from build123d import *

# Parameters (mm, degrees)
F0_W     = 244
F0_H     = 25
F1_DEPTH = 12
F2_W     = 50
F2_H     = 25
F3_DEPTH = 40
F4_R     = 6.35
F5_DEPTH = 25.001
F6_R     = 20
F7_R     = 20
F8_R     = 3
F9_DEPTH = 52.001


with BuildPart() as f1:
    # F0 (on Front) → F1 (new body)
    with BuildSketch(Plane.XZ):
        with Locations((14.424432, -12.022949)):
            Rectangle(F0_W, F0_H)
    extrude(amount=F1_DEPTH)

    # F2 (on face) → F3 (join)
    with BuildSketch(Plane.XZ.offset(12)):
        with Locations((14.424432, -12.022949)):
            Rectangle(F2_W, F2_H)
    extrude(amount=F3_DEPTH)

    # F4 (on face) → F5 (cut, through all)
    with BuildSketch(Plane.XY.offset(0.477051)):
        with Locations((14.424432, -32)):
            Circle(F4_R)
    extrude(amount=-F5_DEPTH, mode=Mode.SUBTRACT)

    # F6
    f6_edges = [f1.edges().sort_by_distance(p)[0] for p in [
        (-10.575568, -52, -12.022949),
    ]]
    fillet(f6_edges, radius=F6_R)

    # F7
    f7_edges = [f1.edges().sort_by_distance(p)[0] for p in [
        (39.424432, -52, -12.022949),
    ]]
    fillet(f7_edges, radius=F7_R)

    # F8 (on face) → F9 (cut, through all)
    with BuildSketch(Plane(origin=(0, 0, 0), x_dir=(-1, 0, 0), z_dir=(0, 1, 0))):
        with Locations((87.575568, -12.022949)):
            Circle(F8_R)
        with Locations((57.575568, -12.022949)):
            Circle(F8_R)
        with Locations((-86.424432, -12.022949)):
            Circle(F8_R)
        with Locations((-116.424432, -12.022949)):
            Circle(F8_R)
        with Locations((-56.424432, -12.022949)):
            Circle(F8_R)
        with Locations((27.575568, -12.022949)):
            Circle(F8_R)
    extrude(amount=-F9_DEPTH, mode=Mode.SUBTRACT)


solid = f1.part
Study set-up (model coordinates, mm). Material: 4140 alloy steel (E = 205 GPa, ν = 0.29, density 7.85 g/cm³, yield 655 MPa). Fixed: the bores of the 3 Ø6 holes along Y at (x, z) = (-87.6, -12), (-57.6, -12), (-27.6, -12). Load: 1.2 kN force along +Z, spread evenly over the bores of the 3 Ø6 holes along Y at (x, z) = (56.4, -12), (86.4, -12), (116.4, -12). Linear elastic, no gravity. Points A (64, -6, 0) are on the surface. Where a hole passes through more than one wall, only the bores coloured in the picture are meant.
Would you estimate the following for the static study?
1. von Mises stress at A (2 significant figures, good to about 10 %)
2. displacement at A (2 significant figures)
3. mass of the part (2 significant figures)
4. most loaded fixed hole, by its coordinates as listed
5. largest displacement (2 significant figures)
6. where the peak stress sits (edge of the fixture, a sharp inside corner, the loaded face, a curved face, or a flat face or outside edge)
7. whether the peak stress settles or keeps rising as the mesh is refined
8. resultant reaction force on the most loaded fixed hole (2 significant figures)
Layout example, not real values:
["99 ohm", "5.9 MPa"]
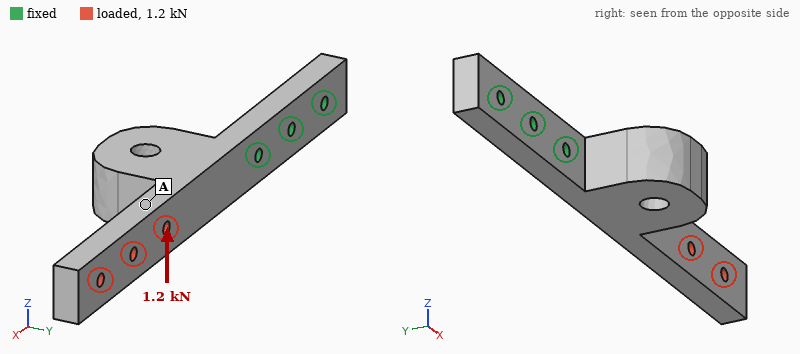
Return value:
["22 MPa", "0.15 mm", "890 g", "(-27.6, -12)", "0.33 mm", "edge of the fixture", "keeps rising", "4.1 kN"]
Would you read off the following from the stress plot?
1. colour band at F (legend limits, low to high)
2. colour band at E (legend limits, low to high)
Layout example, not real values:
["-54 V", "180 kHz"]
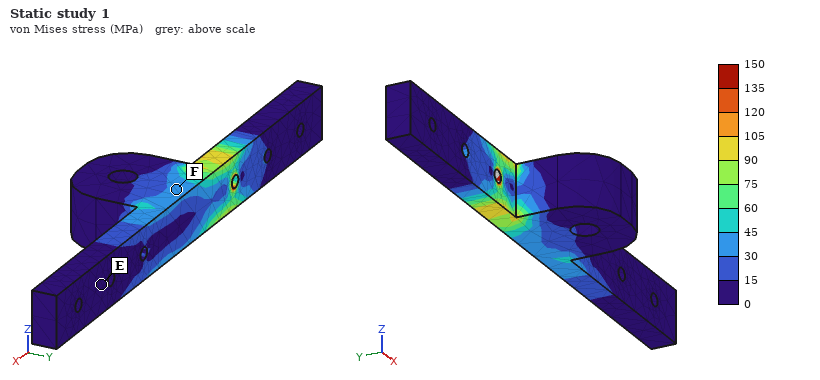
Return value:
["30 to 45 MPa", "0 to 15 MPa"]
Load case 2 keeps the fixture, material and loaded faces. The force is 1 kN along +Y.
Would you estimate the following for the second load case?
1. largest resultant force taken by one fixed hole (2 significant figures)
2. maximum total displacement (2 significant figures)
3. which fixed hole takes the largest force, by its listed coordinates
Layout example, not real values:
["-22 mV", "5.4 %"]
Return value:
["1.9 kN", "0.72 mm", "(-27.6, -12)"]
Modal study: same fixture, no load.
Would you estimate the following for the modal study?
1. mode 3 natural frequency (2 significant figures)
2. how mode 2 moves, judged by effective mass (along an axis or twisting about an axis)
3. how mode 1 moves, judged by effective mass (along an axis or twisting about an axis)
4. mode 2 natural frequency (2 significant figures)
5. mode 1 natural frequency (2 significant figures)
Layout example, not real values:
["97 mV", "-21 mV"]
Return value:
["1700 Hz", "along Z", "along Y", "710 Hz", "440 Hz"]
